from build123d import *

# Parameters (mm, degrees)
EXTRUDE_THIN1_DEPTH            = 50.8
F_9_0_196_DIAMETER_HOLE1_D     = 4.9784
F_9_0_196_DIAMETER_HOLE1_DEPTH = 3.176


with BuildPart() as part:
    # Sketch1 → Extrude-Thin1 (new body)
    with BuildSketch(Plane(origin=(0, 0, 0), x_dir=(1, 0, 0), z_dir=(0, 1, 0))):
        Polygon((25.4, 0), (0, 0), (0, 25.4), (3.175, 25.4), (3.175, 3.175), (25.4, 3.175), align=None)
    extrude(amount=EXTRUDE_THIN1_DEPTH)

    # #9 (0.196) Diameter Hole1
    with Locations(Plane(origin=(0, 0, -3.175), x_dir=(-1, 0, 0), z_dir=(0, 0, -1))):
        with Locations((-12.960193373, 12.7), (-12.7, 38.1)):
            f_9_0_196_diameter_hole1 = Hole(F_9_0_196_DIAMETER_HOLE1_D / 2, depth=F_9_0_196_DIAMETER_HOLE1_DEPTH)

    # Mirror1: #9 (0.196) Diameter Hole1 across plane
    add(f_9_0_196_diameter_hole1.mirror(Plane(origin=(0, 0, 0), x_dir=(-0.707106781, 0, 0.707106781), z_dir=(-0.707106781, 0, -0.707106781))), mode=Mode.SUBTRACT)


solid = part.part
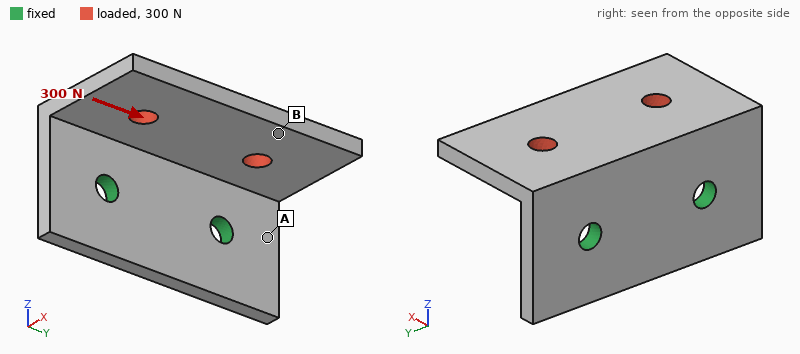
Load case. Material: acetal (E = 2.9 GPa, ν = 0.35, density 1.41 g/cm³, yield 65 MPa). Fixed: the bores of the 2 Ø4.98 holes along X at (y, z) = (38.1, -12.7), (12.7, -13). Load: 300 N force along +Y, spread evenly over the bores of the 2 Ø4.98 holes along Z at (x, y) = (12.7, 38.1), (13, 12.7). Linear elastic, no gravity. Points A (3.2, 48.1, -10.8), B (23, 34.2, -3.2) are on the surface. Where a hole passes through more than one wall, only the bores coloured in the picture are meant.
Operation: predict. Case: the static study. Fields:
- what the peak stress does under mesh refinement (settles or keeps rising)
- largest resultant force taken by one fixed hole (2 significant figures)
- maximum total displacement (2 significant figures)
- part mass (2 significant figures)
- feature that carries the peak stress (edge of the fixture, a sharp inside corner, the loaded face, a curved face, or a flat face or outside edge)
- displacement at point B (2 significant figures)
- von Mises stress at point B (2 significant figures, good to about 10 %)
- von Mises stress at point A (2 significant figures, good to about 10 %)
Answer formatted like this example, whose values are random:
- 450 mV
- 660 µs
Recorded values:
- keeps rising
- 220 N
- 0.58 mm
- 10 g
- edge of the fixture
- 0.36 mm
- 2.6 MPa
- 8.3 MPa
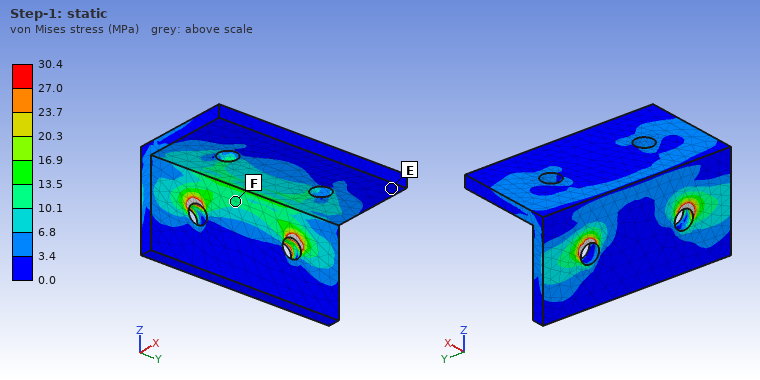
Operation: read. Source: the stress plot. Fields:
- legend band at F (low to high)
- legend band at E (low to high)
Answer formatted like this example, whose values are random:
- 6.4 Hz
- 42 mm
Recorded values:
- 10.1 to 13.5 MPa
- 0.0 to 3.4 MPa
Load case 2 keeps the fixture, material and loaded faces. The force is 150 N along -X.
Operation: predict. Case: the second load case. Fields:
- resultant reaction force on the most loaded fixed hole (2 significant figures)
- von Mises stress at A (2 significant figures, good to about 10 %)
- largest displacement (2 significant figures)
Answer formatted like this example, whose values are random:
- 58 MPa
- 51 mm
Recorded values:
- 76 N
- 6.5 MPa
- 0.57 mm
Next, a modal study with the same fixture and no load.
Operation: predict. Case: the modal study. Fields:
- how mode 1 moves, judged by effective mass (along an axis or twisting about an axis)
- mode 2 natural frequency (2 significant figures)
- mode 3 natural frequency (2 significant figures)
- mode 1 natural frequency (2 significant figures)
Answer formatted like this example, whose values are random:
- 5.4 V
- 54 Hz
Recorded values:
- along Z
- 1300 Hz
- 2100 Hz
- 780 Hz
